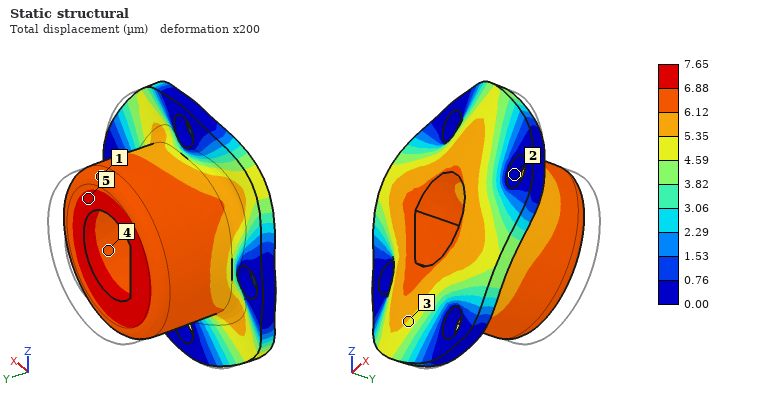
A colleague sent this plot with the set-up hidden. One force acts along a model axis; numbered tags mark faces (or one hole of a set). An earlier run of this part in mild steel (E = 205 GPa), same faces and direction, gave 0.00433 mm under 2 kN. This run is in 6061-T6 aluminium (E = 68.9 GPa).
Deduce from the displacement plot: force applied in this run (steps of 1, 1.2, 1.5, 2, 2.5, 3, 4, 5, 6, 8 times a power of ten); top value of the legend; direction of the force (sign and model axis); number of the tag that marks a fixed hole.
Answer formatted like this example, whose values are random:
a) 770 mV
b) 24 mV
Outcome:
a) 1.2 kN
b) 7.65 µm
c) -Y
d) 2
